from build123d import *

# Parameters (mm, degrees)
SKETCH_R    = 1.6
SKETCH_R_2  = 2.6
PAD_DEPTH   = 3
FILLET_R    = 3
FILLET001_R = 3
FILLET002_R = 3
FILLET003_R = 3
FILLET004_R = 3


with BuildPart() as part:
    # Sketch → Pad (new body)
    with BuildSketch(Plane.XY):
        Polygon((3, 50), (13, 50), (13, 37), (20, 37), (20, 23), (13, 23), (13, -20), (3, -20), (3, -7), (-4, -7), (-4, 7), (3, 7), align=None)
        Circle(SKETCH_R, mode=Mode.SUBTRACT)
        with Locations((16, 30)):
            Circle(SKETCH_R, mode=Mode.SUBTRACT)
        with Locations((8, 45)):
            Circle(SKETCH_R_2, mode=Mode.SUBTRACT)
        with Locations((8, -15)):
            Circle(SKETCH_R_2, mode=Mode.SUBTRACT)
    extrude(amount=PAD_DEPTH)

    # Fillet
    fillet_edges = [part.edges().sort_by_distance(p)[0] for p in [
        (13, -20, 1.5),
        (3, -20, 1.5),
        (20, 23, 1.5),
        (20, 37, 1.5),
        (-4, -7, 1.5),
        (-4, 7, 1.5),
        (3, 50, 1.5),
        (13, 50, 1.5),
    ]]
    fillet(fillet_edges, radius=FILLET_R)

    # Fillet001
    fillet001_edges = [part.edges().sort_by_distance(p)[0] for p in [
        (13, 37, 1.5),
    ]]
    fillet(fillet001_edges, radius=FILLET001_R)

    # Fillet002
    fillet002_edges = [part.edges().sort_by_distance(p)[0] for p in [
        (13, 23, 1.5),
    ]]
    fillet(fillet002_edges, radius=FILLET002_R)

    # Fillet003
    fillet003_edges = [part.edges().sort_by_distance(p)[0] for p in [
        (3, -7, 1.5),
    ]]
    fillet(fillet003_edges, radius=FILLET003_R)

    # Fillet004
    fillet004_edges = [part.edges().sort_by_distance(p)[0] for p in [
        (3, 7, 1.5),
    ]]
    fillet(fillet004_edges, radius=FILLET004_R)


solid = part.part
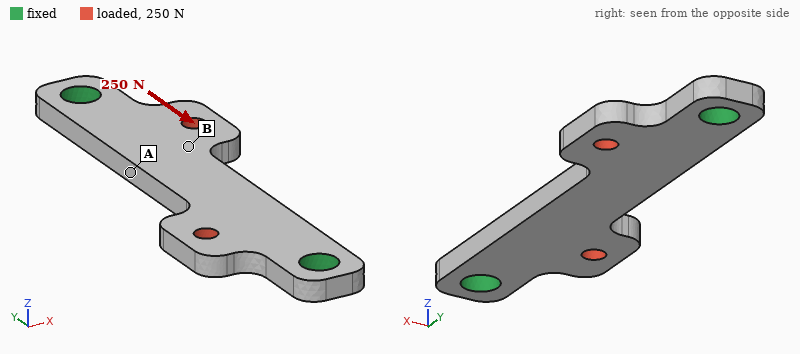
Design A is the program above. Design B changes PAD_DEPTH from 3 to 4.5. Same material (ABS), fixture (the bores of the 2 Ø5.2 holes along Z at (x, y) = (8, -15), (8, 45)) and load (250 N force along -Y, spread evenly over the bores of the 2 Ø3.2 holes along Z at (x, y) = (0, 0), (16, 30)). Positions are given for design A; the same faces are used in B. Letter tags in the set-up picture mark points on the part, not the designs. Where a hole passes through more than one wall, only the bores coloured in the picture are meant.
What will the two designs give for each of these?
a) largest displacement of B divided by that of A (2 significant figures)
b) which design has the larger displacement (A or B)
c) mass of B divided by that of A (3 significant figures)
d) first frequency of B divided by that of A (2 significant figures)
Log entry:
0.67
A
1.50
1.4
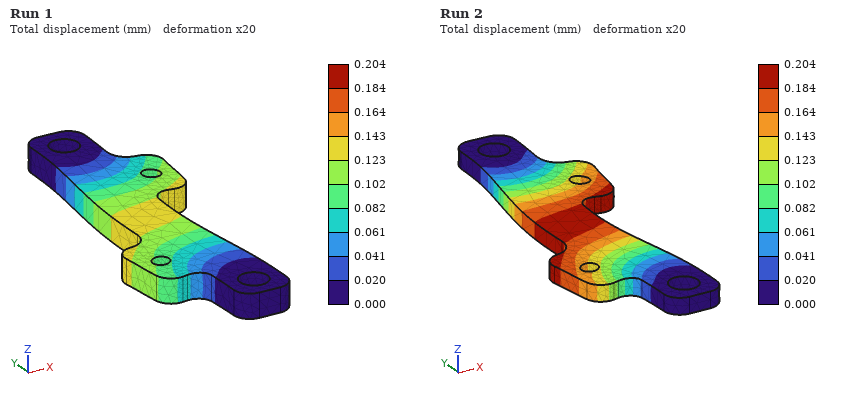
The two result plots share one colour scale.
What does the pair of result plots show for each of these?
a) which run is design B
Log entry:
Run 1
